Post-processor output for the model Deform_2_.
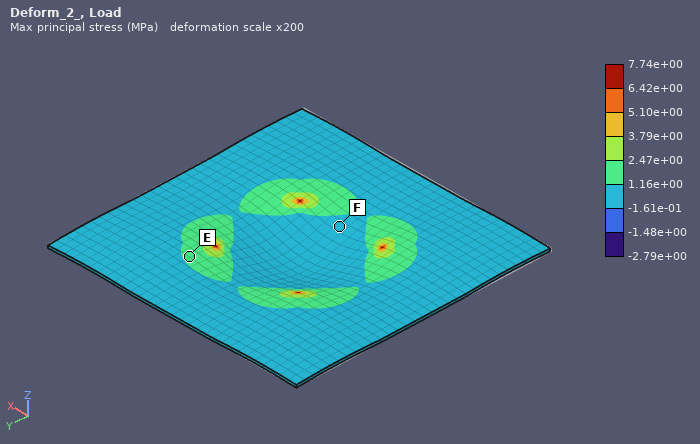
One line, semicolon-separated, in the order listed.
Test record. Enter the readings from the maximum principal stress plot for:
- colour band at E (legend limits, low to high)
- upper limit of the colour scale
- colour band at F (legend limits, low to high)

1.16e+00 to 2.47e+00 MPa; 7.74e+00 MPa; -1.61e-01 to 1.16e+00 MPa
